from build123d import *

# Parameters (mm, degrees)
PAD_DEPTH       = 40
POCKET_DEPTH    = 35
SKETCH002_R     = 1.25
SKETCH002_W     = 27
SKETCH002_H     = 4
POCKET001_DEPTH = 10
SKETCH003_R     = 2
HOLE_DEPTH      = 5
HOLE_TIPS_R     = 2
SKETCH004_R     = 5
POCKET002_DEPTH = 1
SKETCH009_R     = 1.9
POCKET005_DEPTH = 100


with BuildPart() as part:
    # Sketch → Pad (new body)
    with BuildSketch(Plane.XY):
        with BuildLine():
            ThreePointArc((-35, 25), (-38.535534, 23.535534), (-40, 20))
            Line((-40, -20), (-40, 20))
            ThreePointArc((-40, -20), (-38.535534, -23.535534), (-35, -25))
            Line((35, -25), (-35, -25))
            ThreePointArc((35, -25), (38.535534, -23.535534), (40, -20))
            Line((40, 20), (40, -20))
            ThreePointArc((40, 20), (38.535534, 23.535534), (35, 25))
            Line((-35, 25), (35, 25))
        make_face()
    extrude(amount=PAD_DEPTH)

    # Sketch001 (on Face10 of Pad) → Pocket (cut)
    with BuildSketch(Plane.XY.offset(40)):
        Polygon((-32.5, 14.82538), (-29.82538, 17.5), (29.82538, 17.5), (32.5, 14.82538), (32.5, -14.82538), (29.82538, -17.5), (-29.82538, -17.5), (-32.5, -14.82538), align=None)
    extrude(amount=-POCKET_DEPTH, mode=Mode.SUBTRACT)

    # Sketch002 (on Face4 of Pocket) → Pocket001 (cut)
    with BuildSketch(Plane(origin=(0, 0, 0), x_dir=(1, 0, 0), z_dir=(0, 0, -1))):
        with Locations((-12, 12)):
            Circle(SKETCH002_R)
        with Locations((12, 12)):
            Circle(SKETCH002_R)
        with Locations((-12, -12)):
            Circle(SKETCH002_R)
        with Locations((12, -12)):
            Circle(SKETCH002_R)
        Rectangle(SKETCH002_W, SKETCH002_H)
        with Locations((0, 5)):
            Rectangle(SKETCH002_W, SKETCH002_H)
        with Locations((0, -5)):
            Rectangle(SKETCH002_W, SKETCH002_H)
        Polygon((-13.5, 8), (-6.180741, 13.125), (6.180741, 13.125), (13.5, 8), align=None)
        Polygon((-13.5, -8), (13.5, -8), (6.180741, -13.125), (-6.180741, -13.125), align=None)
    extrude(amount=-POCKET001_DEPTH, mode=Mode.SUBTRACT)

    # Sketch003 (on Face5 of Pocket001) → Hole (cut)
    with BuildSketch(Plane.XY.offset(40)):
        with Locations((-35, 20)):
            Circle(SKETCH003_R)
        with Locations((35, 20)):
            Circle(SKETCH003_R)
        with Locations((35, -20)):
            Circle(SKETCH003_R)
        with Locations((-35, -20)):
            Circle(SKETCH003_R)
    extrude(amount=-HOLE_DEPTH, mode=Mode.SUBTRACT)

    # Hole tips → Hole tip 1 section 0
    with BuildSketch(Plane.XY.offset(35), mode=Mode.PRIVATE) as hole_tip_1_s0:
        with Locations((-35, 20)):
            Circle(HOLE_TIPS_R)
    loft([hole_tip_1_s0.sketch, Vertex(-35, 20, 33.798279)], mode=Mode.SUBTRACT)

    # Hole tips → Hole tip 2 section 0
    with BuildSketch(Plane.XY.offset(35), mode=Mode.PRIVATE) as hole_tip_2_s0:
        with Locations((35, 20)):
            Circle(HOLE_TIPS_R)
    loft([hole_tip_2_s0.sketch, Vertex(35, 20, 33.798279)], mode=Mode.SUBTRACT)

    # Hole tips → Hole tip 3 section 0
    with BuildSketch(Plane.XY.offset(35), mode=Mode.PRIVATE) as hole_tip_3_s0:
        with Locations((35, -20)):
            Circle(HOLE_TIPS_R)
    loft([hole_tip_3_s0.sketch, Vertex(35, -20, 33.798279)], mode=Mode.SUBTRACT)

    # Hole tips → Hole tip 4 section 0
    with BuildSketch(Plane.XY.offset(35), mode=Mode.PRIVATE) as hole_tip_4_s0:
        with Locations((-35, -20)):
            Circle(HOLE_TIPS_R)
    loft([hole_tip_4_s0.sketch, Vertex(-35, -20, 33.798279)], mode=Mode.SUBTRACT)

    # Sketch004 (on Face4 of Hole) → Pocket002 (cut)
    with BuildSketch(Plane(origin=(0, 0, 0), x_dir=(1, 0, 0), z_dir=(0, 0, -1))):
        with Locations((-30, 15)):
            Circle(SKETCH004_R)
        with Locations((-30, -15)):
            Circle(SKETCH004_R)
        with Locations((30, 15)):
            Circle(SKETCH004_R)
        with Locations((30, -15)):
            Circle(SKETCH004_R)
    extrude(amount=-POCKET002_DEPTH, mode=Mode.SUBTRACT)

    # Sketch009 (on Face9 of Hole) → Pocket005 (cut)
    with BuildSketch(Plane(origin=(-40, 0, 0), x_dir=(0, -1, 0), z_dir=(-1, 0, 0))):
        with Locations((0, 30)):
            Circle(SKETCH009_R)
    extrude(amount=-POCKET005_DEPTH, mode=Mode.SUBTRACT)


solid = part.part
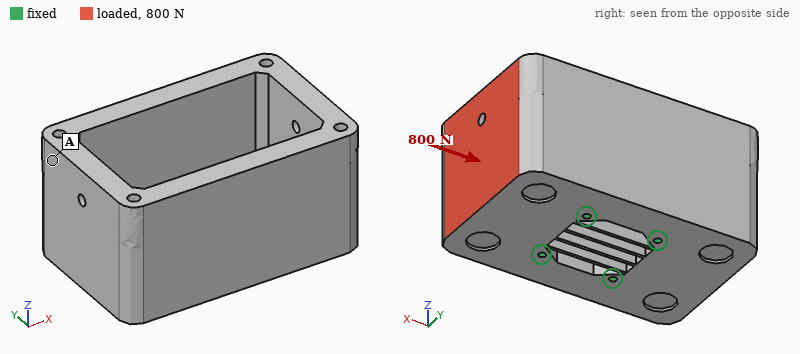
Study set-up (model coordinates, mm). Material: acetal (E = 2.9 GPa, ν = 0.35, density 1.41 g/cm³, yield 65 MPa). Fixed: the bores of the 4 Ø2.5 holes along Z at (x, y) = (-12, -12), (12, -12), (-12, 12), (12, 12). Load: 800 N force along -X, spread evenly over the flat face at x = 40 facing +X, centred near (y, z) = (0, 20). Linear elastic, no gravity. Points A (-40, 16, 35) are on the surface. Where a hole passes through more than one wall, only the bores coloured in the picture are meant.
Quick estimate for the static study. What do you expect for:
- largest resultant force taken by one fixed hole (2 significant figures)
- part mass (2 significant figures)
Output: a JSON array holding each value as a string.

["360 N", "110 g"]
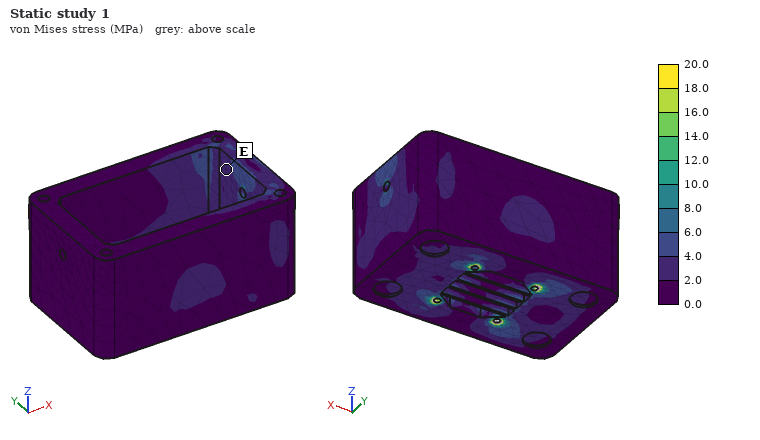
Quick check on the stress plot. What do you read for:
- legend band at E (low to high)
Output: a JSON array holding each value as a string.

["2.0 to 4.0 MPa"]
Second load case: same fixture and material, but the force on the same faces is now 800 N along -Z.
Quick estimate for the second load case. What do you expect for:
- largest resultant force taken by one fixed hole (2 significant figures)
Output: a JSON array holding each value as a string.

["770 N"]
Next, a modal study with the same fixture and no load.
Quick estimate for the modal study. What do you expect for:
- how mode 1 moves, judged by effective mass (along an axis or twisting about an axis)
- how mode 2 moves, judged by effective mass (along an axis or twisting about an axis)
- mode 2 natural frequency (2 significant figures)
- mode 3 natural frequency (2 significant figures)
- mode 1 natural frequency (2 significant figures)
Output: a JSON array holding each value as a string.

["along X", "along Y", "810 Hz", "1200 Hz", "760 Hz"]
